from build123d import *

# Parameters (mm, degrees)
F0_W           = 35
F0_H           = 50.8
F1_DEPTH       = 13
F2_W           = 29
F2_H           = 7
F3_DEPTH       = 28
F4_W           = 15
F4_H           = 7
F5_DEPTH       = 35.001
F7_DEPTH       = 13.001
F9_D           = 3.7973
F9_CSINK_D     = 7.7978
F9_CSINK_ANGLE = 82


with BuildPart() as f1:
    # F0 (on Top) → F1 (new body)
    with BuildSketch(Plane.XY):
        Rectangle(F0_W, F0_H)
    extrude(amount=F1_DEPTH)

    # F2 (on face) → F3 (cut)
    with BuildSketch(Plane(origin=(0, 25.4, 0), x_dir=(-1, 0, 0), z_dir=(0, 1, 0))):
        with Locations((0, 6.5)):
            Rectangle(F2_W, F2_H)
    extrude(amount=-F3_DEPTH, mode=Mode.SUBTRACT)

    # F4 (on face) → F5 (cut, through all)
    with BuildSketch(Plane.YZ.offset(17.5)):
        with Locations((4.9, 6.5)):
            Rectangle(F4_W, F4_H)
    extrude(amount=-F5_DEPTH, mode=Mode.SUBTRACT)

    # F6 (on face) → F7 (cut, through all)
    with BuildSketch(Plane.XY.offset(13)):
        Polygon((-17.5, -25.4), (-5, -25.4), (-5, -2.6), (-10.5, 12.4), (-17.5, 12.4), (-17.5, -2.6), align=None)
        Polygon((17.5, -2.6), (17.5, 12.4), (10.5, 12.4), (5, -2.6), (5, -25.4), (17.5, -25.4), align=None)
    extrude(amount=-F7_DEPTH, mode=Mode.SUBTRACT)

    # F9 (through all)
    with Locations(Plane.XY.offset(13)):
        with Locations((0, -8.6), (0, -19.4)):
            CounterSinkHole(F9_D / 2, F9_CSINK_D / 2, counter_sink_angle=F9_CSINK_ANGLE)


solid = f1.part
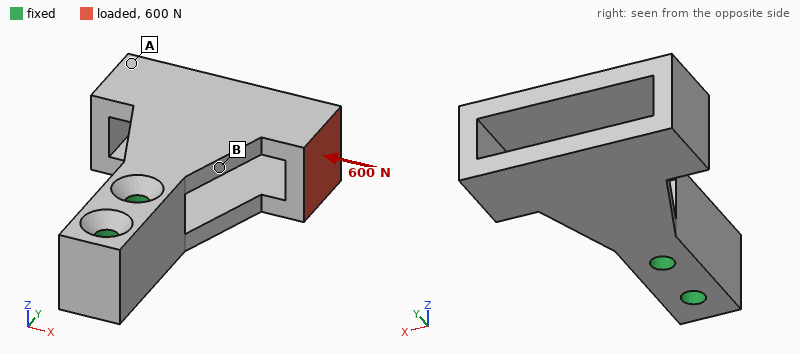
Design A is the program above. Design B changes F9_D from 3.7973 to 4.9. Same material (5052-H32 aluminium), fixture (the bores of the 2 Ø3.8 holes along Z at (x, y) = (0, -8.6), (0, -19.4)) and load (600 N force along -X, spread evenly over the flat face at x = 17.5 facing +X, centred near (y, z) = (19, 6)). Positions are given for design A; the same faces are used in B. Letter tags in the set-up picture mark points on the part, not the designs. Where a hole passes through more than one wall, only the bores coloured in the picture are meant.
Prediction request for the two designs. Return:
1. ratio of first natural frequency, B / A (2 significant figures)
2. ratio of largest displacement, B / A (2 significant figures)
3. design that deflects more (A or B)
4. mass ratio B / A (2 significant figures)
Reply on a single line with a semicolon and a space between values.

1.0; 0.91; A; 0.98
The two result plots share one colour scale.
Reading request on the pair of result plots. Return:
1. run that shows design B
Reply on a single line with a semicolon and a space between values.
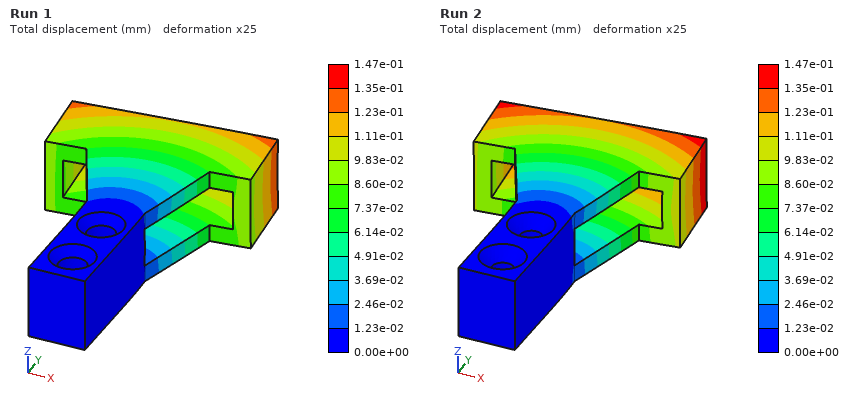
Run 1
